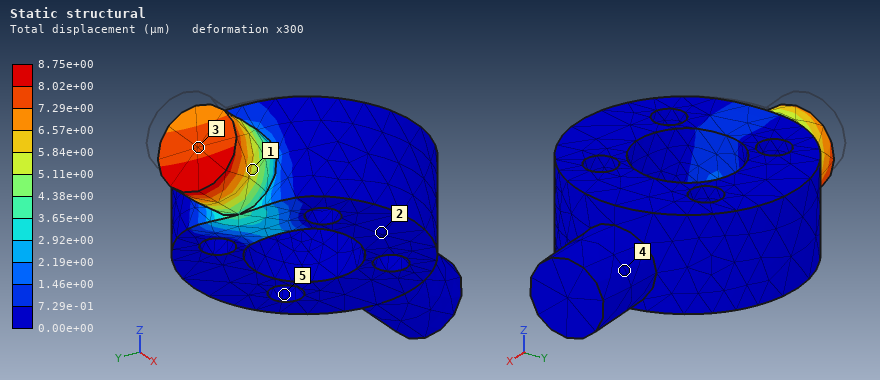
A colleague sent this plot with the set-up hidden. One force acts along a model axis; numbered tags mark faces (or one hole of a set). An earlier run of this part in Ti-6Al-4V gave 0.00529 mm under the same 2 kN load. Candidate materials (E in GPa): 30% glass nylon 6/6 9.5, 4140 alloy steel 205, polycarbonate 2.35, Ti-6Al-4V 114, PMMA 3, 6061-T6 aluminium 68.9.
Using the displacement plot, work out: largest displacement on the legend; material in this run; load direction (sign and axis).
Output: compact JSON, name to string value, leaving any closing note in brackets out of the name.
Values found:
{"largest displacement on the legend": "8.75e+00 µm", "material in this run": "6061-T6 aluminium", "load direction": "+X"}
